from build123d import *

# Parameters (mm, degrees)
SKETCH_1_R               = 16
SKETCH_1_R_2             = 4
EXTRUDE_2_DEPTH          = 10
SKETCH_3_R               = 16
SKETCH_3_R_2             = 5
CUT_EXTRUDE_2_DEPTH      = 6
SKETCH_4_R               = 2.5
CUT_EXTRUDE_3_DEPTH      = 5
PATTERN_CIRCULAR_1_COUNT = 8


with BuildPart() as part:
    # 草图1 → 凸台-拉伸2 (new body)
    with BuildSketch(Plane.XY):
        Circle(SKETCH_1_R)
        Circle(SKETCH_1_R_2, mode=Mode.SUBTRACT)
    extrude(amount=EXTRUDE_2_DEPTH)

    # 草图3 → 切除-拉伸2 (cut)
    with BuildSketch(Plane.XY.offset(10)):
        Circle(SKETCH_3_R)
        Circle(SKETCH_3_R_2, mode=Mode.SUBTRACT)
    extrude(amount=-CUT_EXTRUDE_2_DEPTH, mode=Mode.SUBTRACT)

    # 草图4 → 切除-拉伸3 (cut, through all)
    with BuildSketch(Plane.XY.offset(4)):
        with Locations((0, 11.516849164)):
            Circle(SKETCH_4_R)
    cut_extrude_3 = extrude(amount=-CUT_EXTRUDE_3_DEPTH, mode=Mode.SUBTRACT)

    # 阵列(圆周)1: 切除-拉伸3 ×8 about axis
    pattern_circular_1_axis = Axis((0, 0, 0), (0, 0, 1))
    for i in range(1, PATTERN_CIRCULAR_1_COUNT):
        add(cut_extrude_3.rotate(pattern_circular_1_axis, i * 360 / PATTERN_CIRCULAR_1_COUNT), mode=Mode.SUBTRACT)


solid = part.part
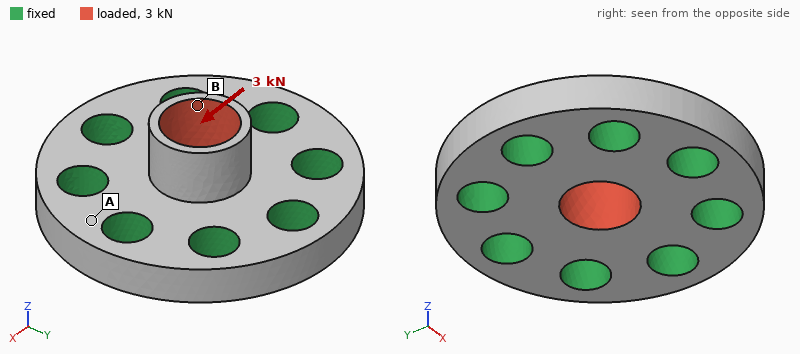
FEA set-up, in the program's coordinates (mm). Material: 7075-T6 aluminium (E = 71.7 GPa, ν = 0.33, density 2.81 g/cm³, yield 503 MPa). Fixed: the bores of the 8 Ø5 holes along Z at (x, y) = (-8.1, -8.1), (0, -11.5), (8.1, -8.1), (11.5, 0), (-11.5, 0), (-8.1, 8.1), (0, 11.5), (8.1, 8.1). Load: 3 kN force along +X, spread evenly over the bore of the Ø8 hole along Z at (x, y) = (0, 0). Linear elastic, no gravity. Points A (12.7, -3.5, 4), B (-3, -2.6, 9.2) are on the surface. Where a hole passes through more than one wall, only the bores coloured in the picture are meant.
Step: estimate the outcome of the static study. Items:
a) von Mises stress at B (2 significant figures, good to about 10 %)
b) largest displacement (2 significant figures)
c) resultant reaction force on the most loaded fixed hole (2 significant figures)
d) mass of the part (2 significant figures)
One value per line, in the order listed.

60 MPa
29 µm
710 N
7.2 g
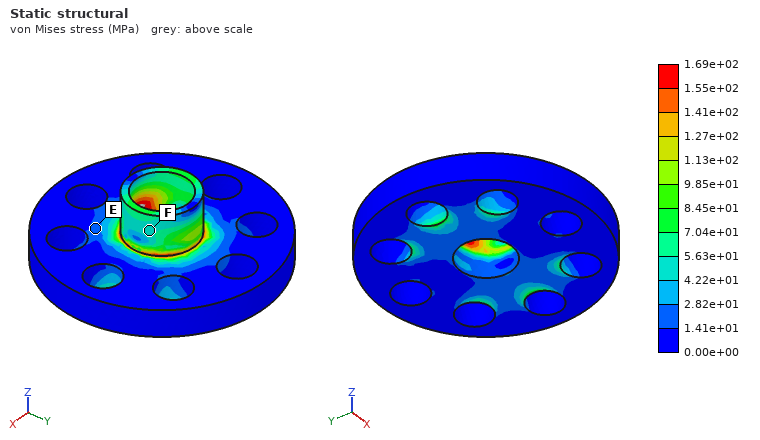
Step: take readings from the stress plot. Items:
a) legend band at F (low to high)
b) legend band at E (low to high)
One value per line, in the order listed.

4.22e+01 to 5.63e+01 MPa
1.41e+01 to 2.82e+01 MPa
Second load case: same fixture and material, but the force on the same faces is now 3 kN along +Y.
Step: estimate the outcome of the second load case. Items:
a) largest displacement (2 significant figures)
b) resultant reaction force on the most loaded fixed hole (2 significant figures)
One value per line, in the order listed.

29 µm
710 N
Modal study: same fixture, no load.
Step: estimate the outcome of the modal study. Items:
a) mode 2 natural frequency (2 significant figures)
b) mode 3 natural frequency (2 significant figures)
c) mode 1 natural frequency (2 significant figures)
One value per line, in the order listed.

58 kHz
66 kHz
58 kHz
